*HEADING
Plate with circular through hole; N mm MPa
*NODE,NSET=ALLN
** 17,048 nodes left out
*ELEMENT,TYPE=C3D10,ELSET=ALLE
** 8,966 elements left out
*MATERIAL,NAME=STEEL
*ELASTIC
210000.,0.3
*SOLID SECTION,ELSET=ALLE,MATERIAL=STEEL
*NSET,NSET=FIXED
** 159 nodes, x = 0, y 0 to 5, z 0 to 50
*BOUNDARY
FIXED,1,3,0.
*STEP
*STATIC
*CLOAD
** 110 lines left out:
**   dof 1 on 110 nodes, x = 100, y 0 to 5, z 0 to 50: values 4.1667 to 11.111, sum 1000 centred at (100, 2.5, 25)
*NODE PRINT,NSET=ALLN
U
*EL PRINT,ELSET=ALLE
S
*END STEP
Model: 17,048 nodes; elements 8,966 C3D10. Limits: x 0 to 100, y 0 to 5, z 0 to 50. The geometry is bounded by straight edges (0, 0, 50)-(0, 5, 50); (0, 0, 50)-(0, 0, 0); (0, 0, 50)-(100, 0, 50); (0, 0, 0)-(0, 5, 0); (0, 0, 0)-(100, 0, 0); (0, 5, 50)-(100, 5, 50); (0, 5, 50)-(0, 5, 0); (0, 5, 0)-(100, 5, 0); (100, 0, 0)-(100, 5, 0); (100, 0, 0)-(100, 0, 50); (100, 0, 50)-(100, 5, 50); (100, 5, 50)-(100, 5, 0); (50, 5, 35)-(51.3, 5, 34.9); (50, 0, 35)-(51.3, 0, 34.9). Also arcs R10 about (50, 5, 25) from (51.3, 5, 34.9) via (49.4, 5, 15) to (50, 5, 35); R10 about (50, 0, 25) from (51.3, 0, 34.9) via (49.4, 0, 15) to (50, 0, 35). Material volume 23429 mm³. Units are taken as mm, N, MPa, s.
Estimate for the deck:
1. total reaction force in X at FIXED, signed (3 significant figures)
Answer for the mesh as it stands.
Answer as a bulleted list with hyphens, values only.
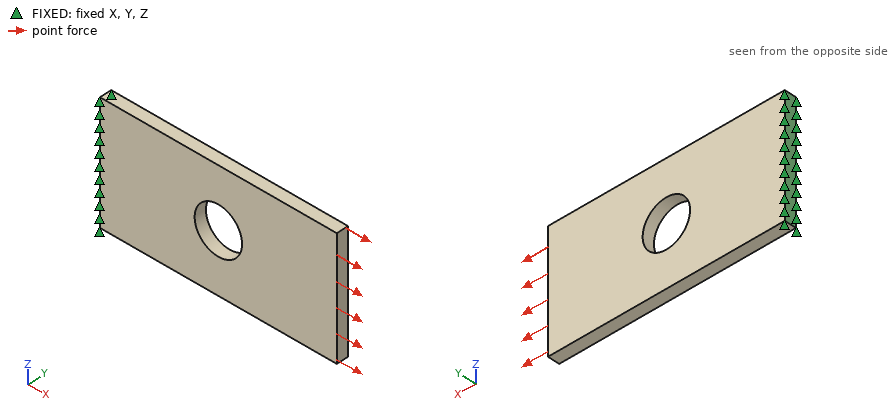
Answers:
- -1000 N
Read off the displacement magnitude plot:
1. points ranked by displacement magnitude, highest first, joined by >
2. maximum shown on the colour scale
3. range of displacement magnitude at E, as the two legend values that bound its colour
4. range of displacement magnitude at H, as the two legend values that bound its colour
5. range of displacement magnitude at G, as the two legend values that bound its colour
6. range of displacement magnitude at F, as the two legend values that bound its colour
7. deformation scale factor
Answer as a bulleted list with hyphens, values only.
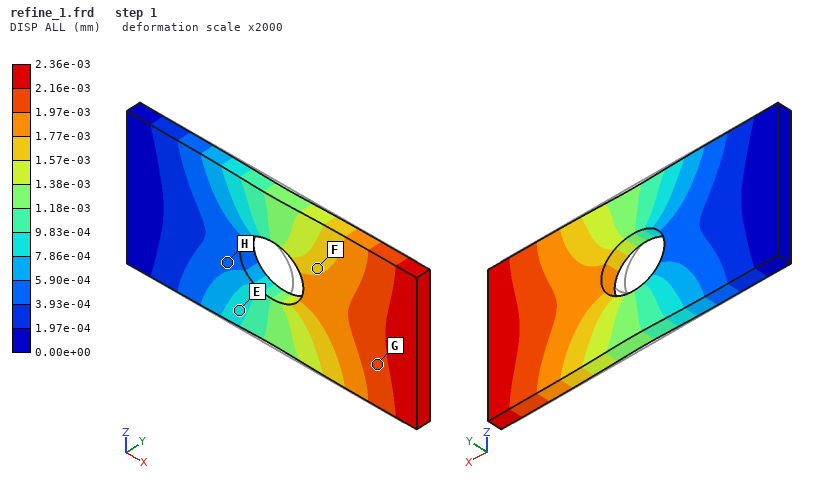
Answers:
- G > F > E > H
- 2.36e-03 mm
- 7.86e-04 to 9.83e-04 mm
- 3.93e-04 to 5.90e-04 mm
- 1.97e-03 to 2.16e-03 mm
- 1.57e-03 to 1.77e-03 mm
- 2000
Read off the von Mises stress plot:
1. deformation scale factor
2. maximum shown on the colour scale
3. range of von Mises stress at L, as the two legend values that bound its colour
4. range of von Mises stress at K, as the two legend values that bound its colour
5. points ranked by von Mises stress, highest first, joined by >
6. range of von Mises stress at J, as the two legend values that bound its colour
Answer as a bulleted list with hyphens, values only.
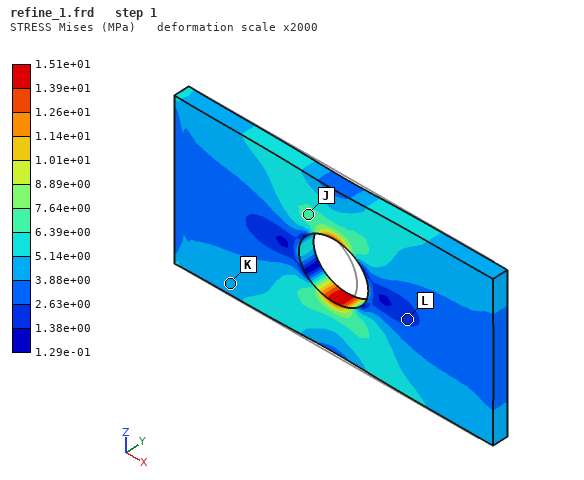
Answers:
- 2000
- 1.51e+01 MPa
- 1.38e+00 to 2.63e+00 MPa
- 3.88e+00 to 5.14e+00 MPa
- J > K > L
- 6.39e+00 to 7.64e+00 MPa
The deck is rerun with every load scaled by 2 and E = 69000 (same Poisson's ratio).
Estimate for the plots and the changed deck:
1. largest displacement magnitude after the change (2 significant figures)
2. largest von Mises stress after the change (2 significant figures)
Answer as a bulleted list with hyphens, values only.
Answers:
- 0.014 mm
- 30 MPa
